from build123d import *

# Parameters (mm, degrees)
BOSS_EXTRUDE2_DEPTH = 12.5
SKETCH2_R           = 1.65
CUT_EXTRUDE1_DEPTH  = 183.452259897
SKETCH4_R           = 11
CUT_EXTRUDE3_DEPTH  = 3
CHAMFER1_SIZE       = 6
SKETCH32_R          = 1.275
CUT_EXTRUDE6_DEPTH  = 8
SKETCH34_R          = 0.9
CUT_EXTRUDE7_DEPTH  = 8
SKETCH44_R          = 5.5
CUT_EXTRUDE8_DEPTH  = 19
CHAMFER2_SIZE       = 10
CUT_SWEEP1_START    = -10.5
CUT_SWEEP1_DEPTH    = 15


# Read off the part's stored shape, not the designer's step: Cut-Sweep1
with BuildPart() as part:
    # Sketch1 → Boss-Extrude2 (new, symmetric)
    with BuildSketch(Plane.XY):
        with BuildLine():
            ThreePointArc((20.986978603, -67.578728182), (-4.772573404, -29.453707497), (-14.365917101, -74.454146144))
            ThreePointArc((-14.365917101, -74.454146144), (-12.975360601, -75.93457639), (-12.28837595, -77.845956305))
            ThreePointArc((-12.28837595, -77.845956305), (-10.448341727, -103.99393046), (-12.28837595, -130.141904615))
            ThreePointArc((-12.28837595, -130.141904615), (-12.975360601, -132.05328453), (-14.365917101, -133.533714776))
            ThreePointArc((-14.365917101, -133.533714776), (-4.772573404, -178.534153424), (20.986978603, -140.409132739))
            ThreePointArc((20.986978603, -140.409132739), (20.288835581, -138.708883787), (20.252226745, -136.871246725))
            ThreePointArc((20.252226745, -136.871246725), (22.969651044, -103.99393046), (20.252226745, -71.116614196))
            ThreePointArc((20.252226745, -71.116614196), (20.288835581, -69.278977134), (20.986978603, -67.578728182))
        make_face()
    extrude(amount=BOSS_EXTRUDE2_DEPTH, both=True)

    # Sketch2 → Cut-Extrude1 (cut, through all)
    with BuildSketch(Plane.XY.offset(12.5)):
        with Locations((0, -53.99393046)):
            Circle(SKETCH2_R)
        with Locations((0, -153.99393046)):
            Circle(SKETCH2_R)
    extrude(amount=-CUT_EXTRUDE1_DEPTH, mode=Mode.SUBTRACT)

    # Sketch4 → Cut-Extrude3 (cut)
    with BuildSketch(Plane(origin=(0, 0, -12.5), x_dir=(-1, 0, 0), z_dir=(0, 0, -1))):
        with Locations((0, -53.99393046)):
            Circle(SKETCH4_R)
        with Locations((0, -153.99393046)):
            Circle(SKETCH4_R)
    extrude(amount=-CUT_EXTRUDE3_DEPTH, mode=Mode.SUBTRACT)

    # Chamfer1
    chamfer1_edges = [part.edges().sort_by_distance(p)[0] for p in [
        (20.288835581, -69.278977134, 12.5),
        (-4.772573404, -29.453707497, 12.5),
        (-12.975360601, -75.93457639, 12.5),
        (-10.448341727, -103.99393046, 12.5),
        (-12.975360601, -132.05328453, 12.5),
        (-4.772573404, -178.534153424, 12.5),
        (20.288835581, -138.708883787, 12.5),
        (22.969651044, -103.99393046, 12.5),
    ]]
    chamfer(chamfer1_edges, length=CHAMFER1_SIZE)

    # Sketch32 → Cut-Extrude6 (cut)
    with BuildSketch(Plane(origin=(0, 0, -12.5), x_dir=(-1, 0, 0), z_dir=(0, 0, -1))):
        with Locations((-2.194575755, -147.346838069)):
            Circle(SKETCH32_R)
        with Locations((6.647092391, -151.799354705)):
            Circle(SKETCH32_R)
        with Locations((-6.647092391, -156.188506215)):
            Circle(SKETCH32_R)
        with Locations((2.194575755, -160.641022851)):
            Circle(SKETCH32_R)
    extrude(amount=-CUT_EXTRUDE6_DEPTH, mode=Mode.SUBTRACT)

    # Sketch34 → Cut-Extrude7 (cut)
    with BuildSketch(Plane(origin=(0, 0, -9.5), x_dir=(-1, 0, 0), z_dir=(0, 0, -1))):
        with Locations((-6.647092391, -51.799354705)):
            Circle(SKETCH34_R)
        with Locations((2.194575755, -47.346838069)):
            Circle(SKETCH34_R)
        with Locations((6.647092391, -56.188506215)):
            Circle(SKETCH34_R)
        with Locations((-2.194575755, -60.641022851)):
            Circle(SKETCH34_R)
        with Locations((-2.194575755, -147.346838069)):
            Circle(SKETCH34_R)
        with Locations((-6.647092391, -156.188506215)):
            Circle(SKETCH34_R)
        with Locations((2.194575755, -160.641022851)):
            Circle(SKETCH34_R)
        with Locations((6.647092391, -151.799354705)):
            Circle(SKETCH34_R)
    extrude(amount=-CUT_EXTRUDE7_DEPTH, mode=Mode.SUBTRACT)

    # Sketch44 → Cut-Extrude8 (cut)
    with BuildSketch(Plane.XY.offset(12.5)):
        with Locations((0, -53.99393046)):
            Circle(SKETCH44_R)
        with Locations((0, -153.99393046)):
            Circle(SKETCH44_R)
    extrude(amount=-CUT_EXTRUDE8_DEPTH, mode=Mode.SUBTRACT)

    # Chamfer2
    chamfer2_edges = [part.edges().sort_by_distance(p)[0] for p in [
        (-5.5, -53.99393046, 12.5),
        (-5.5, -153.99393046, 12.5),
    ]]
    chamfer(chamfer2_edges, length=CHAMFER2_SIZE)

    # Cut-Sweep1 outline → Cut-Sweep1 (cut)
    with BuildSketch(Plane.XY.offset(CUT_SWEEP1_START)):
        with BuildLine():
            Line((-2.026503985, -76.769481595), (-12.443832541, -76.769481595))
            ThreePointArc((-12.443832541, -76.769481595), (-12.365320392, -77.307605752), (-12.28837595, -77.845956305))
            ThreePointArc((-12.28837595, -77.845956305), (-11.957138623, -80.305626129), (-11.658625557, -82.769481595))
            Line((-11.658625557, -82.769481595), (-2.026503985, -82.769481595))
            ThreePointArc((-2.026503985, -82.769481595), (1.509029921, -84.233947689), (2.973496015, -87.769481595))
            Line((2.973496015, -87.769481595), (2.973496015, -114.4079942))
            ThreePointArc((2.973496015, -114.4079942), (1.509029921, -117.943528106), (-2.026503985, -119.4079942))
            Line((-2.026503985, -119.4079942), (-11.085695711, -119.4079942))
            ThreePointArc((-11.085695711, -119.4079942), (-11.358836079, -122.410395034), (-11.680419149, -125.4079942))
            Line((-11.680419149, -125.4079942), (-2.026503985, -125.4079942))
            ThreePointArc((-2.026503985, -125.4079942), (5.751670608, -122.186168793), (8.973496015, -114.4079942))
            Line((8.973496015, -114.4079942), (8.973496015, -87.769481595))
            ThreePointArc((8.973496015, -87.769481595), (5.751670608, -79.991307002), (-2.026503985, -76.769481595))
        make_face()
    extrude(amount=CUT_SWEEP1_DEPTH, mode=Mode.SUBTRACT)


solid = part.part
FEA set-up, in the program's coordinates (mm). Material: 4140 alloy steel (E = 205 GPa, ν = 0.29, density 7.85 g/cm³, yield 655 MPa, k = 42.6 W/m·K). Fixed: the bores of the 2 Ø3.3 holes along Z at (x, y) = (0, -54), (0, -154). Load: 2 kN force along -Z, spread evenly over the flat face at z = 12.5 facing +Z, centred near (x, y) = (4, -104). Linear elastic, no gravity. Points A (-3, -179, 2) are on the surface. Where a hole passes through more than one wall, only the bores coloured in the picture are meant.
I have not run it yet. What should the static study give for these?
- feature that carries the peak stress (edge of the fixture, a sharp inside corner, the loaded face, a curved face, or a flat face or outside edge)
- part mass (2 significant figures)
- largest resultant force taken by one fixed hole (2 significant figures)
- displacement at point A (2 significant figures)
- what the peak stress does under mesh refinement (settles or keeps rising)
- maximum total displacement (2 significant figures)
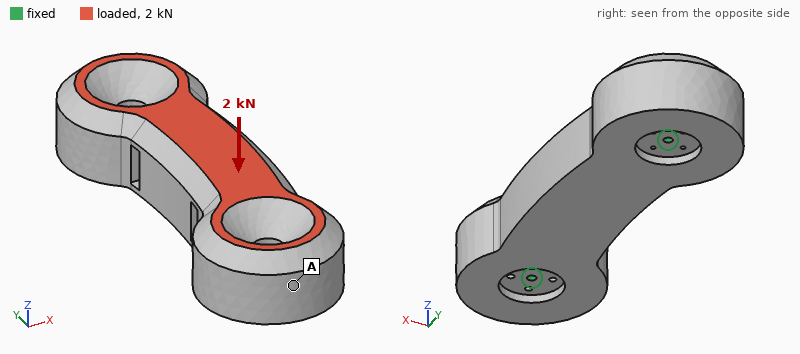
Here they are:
edge of the fixture
940 g
1.1 kN
7.1 µm
keeps rising
24 µm
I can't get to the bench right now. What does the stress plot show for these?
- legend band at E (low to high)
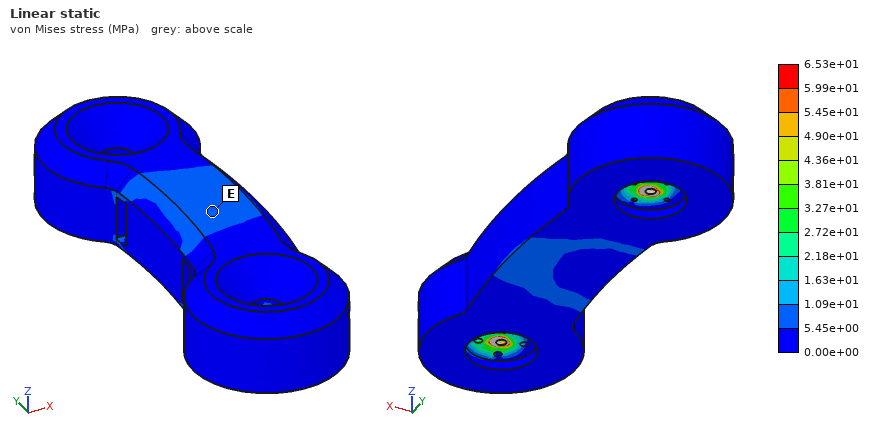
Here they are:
5.45e+00 to 1.09e+01 MPa
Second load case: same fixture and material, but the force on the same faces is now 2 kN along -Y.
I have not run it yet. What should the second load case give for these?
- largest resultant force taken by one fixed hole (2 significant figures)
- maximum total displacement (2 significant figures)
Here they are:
1.1 kN
2.7 µm
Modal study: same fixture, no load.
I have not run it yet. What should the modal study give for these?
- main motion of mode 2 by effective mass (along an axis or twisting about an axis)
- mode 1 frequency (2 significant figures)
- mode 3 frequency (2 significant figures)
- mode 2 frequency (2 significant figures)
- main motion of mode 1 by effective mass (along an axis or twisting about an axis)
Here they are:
along Z
1000 Hz
5300 Hz
4300 Hz
along X
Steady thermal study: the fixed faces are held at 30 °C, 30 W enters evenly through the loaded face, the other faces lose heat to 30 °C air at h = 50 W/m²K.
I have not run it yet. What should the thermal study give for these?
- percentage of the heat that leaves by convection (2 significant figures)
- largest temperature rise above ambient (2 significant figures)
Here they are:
58 %
23 K
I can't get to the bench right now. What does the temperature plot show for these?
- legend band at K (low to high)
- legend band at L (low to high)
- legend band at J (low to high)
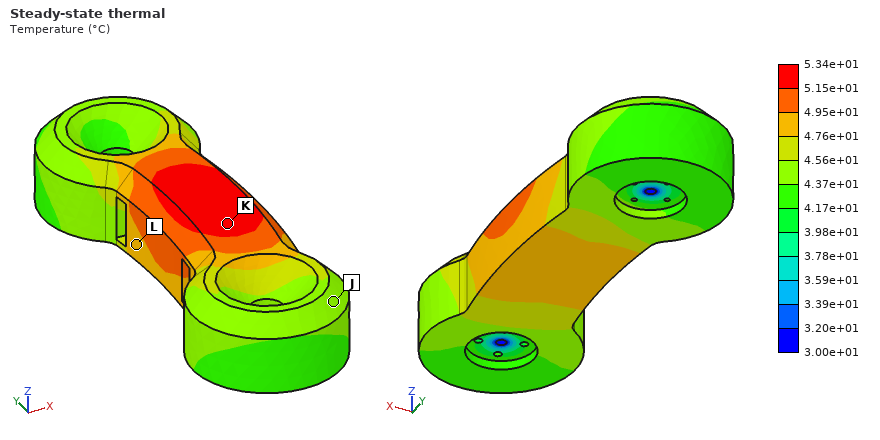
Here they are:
5.15e+01 to 5.34e+01 °C
4.76e+01 to 4.95e+01 °C
4.37e+01 to 4.56e+01 °C
